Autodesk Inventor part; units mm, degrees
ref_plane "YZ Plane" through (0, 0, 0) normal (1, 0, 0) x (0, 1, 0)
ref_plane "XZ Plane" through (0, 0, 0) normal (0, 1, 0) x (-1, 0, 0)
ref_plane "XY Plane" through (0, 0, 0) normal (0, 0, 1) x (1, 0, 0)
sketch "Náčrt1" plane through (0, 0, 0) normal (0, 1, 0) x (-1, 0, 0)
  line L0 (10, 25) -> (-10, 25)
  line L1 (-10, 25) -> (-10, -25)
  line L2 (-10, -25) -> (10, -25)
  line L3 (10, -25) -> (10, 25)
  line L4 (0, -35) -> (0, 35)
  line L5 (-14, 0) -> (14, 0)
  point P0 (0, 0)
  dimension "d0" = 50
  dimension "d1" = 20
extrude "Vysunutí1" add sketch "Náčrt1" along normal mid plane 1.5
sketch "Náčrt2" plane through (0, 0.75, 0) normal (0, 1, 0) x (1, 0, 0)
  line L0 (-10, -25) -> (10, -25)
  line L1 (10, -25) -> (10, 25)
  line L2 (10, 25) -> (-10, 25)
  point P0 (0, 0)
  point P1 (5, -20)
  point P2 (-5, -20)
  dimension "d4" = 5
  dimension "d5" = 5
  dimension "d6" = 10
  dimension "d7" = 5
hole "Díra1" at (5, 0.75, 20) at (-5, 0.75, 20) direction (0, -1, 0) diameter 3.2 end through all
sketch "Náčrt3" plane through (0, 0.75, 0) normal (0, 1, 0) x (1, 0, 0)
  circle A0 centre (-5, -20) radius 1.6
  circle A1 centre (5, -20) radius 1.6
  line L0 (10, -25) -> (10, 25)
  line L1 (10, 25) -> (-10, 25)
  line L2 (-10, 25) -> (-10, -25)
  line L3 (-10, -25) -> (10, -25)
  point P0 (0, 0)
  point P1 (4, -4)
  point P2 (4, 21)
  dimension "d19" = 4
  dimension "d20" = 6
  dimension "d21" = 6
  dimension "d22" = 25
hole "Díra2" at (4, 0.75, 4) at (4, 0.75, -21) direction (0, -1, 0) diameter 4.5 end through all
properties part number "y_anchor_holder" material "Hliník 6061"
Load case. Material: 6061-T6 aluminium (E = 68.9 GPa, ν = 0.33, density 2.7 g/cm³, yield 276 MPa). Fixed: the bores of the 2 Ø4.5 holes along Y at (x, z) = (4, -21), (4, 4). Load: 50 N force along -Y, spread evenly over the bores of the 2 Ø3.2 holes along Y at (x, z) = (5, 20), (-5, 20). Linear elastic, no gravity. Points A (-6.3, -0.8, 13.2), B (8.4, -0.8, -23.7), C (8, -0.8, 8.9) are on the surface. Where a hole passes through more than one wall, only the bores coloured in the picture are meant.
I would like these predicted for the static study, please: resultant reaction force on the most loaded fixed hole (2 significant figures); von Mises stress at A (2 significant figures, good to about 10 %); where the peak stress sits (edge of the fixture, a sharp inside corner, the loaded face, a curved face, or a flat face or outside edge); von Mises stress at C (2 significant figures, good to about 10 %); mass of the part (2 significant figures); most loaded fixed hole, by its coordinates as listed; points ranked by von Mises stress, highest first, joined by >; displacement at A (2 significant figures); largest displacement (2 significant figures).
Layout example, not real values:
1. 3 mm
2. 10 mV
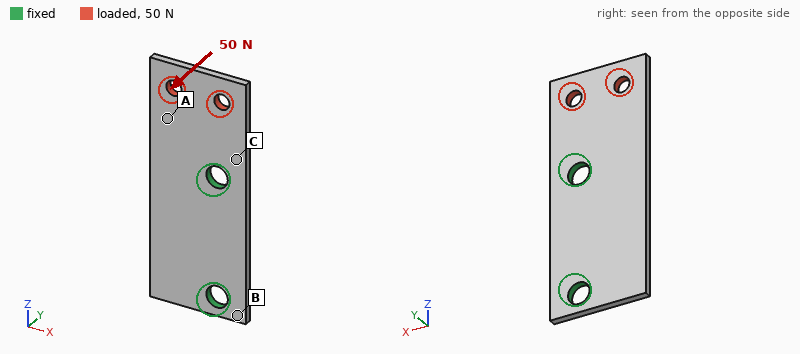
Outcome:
1. 54 N
2. 38 MPa
3. a flat face or outside edge
4. 81 MPa
5. 3.9 g
6. (4, 4)
7. C > A > B
8. 0.083 mm
9. 0.26 mm
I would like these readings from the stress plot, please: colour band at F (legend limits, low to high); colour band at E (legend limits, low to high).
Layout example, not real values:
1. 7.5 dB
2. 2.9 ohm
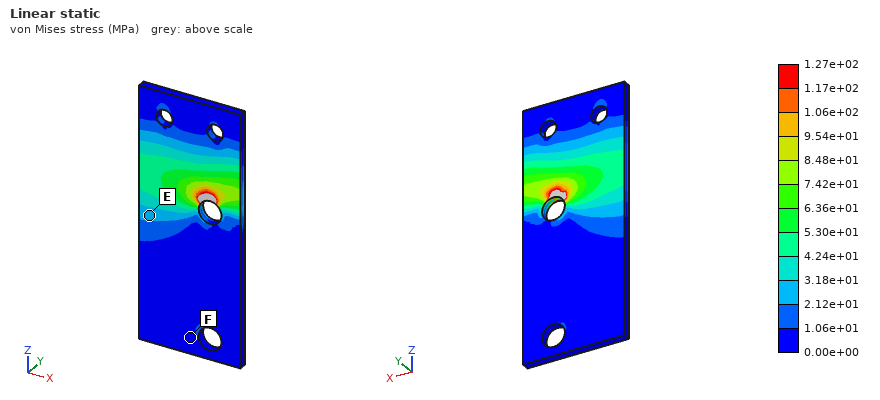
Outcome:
1. 0.00e+00 to 1.06e+01 MPa
2. 2.12e+01 to 3.18e+01 MPa
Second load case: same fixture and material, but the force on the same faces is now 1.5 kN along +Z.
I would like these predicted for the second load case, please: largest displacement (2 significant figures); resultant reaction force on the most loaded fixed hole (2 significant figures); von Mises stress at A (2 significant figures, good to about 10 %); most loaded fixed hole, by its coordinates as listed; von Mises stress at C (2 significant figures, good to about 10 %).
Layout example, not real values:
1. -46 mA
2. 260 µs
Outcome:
1. 28 µm
2. 1.2 kN
3. 49 MPa
4. (4, 4)
5. 37 MPa
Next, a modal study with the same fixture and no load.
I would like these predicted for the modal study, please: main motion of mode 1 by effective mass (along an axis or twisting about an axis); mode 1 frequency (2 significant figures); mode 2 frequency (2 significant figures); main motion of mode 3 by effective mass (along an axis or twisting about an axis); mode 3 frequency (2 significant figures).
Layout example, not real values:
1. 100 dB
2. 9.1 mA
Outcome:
1. along Y
2. 3000 Hz
3. 5600 Hz
4. along Y
5. 7100 Hz
